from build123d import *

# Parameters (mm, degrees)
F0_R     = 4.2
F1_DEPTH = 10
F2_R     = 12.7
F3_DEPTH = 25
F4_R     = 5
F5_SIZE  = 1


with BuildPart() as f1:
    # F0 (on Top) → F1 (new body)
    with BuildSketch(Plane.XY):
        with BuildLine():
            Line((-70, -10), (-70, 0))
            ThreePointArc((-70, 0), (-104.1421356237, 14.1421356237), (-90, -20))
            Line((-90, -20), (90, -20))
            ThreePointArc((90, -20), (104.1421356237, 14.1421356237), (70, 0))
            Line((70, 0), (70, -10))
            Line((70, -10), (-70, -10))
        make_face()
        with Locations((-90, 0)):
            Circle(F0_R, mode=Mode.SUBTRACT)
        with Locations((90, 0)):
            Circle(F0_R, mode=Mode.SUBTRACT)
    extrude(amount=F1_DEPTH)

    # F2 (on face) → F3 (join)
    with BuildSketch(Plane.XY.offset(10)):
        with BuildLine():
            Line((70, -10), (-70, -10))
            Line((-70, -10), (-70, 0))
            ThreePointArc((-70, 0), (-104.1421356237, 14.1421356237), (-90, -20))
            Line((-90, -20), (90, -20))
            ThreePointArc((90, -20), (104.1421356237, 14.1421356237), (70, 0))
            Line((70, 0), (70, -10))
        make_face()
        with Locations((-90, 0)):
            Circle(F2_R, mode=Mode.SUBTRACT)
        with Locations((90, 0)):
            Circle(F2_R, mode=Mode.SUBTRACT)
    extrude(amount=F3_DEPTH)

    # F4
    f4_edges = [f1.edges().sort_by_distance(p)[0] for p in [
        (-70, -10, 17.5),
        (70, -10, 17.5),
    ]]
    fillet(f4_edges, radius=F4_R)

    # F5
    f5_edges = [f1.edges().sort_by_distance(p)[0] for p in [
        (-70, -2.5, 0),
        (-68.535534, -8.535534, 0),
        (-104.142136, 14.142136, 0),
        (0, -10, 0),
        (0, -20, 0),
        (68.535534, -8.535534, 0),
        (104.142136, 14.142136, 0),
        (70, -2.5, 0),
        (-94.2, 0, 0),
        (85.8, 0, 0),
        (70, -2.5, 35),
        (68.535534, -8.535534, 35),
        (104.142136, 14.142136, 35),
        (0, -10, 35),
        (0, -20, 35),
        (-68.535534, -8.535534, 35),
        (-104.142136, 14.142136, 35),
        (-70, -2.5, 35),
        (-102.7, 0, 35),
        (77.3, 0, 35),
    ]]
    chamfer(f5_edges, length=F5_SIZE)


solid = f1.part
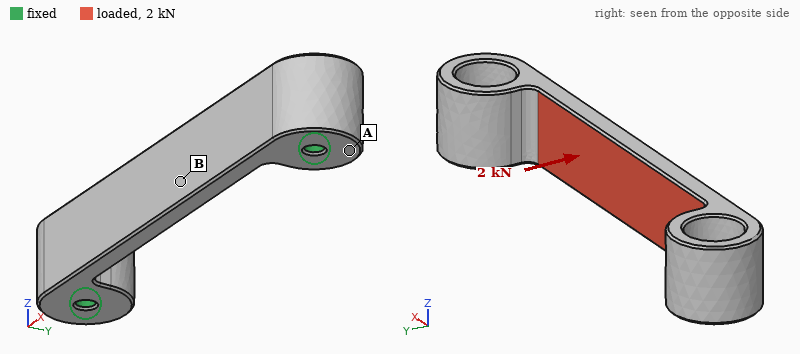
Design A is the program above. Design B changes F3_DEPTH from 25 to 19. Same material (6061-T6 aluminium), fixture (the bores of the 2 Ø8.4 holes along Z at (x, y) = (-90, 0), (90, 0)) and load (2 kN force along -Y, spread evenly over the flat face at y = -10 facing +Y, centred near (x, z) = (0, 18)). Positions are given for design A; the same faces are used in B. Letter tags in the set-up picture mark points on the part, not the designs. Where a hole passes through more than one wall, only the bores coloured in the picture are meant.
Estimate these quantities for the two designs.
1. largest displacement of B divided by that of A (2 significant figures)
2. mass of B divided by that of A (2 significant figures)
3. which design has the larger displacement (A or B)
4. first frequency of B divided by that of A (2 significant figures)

1.1
0.84
B
1.0
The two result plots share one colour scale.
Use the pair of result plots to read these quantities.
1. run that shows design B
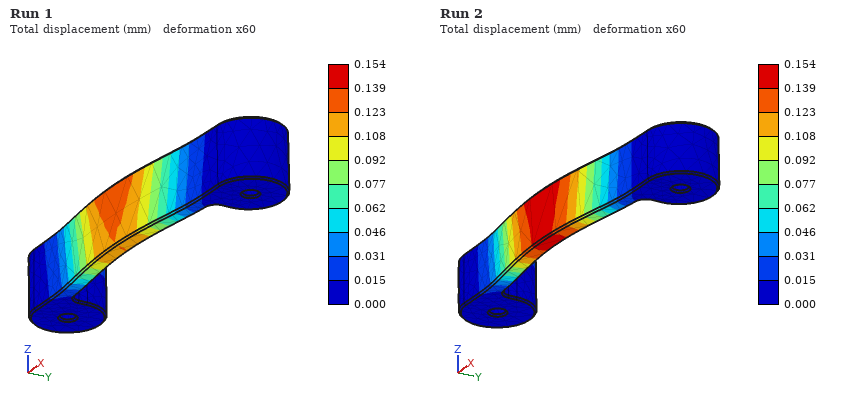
Run 2
